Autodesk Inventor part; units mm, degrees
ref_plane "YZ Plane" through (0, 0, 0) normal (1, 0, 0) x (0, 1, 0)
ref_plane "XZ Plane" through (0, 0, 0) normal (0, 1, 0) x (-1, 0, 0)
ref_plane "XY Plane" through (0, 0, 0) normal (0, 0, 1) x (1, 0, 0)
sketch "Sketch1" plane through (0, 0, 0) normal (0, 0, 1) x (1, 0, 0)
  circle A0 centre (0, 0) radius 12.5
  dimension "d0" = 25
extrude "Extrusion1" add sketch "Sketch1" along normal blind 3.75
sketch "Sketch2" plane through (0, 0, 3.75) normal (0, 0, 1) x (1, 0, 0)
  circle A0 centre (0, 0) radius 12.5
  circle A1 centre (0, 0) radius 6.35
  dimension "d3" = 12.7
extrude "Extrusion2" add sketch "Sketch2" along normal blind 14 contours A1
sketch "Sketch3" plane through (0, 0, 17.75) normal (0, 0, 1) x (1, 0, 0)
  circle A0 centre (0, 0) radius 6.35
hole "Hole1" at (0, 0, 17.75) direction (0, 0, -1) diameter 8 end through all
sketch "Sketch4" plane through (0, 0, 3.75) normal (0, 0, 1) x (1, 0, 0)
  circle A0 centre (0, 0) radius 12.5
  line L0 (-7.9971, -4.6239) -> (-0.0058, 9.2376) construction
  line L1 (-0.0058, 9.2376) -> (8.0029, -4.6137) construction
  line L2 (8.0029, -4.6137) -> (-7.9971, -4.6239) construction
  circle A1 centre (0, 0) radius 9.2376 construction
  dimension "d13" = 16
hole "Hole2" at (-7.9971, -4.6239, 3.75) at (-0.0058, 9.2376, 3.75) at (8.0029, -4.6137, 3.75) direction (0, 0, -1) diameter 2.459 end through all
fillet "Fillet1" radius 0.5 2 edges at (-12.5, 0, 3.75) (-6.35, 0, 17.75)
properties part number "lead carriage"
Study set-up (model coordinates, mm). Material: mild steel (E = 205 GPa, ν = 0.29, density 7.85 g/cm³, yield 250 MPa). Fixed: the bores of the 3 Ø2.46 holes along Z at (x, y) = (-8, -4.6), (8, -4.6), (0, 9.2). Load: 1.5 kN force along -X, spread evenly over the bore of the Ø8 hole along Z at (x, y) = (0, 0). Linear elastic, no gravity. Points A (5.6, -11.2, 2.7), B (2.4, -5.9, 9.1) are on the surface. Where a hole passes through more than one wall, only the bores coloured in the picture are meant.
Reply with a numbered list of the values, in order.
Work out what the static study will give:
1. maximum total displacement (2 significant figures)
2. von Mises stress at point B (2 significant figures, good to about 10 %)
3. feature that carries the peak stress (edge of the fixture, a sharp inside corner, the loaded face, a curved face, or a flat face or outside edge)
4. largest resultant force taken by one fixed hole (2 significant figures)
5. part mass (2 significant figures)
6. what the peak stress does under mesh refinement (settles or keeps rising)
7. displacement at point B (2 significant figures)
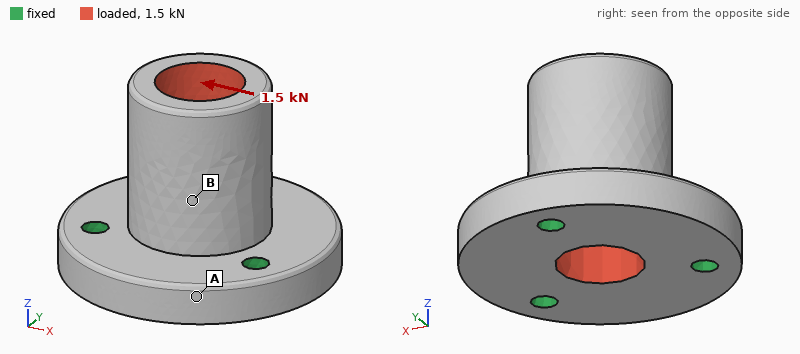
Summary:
1. 9.8 µm
2. 25 MPa
3. edge of the fixture
4. 820 N
5. 21 g
6. keeps rising
7. 4.1 µm
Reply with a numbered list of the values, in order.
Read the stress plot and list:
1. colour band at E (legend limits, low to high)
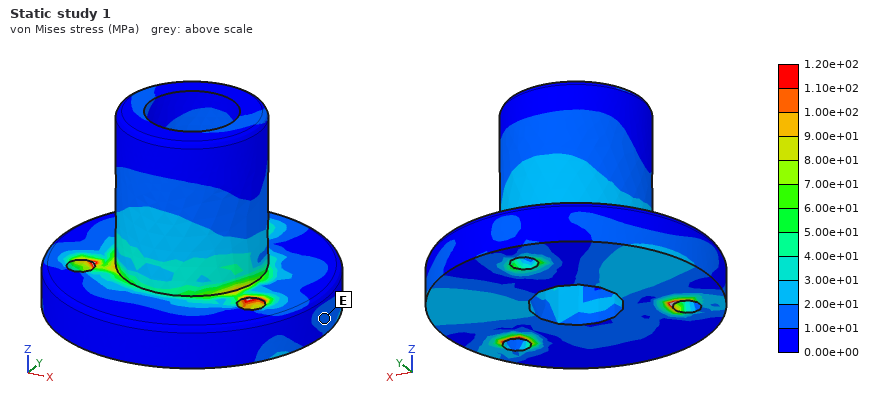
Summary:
1. 1.00e+01 to 2.00e+01 MPa
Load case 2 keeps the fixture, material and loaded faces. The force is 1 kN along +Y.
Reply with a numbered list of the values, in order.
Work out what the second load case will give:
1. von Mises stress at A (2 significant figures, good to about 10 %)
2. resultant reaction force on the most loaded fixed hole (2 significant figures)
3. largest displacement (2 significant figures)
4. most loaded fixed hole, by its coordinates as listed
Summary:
1. 8.2 MPa
2. 610 N
3. 6.6 µm
4. (0, 9.2)
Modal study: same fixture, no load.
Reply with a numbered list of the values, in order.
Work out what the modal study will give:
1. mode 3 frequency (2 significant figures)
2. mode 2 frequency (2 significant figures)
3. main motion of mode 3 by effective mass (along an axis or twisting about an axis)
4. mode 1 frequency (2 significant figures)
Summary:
1. 40 kHz
2. 22 kHz
3. along Z
4. 22 kHz
